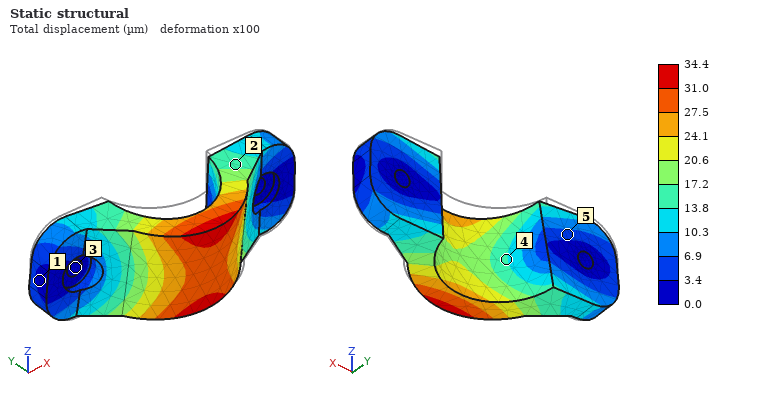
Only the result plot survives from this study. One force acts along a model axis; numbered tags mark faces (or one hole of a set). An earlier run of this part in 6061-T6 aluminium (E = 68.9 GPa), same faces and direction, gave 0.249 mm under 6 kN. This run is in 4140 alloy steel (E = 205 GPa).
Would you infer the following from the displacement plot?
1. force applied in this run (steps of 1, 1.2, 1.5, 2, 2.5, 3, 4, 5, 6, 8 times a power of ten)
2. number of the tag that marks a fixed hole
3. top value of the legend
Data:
2.5 kN
3
34.4 µm
